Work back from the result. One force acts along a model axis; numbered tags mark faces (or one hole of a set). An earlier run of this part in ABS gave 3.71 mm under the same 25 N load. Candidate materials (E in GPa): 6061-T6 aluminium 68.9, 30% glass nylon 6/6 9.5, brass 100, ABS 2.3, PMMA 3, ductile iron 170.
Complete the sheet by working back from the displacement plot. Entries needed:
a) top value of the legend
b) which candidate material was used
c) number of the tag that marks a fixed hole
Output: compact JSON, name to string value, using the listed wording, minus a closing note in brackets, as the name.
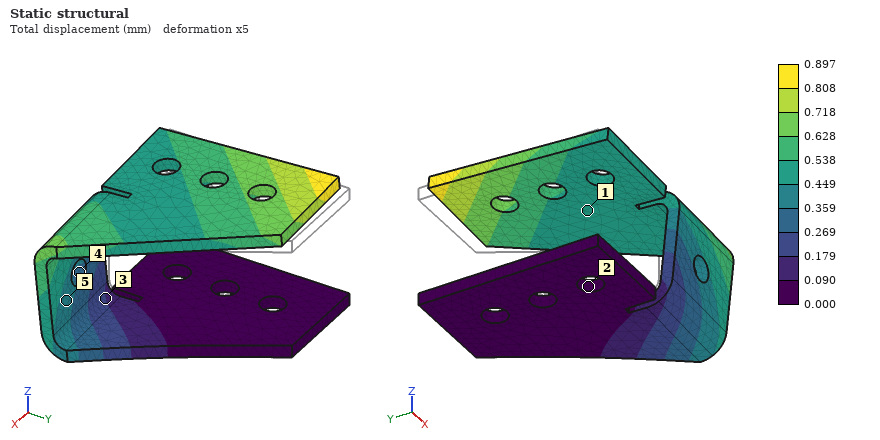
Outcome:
{"top value of the legend": "0.897 mm", "which candidate material was used": "30% glass nylon 6/6", "number of the tag that marks a fixed hole": "2"}
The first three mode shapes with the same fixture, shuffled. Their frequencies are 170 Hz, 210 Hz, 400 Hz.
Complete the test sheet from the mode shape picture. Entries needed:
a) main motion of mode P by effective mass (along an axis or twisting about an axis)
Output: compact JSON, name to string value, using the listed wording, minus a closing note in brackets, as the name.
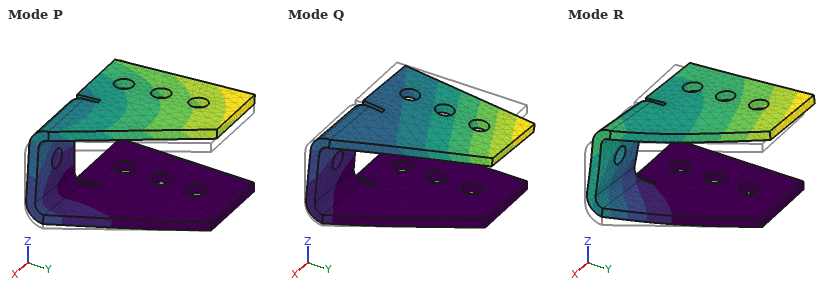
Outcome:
{"main motion of mode P by effective mass": "along X"}
